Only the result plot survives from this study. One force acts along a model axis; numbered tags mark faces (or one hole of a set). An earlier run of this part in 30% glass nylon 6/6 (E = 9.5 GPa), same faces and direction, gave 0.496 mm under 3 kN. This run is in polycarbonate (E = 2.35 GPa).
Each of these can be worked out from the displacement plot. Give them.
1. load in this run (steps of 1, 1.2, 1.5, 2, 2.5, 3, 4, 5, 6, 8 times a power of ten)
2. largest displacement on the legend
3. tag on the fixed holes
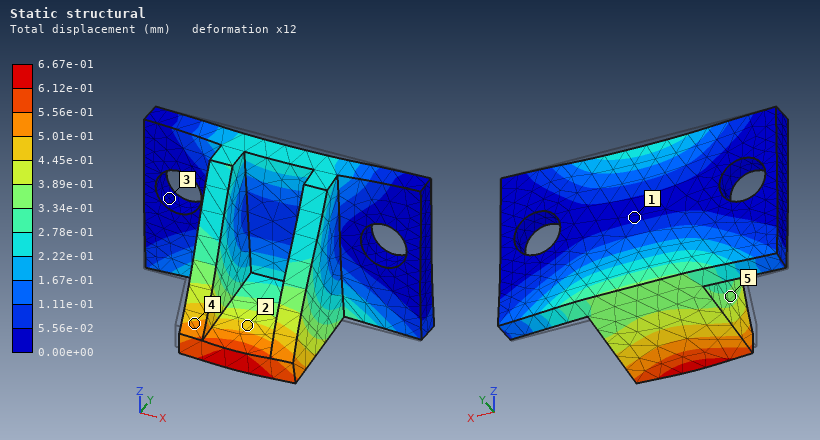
1 kN
6.67e-01 mm
3
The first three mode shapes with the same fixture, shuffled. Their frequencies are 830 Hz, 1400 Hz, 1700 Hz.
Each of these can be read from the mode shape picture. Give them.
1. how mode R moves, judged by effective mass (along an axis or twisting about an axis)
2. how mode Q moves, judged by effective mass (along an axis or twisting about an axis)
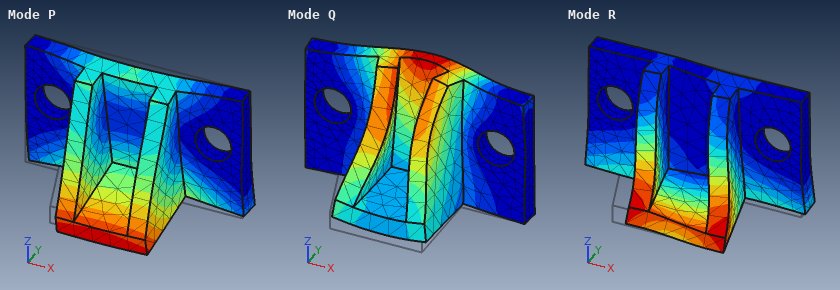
along X
along Y
